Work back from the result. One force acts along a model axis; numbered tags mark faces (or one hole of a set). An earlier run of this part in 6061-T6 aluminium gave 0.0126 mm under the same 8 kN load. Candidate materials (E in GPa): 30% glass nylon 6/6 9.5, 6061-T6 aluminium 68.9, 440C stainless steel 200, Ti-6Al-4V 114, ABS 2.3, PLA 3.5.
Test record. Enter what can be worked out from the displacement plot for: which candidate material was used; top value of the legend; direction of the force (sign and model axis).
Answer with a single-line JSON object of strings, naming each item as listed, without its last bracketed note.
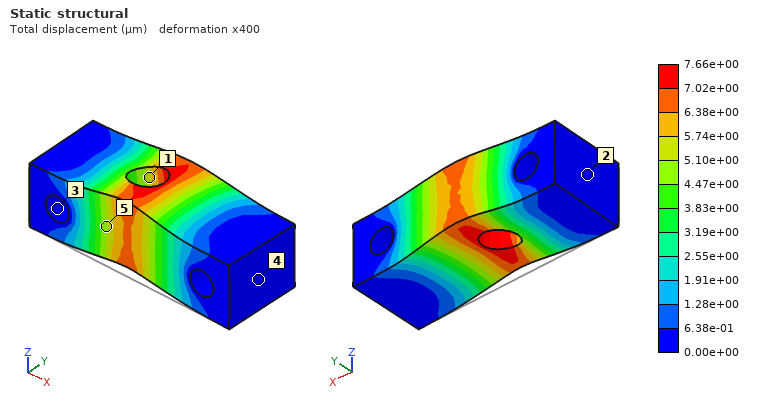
{"which candidate material was used": "Ti-6Al-4V", "top value of the legend": "7.66e+00 µm", "direction of the force": "+Y"}
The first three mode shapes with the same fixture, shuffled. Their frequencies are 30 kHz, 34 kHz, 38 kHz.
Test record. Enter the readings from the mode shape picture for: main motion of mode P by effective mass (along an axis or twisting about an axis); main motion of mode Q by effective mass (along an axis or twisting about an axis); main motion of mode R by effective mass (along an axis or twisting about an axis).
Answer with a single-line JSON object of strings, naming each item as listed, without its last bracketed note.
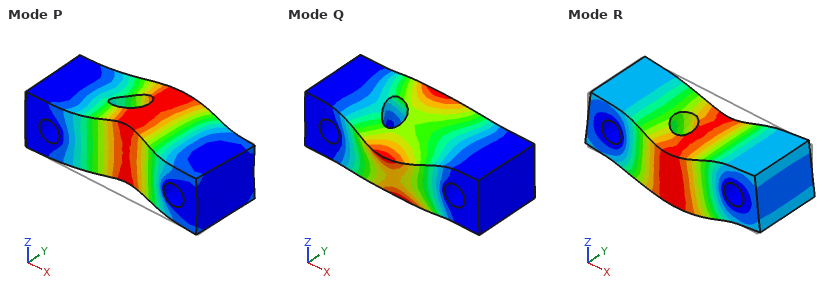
{"main motion of mode P by effective mass": "along Y", "main motion of mode Q by effective mass": "twisting about X", "main motion of mode R by effective mass": "along Z"}
